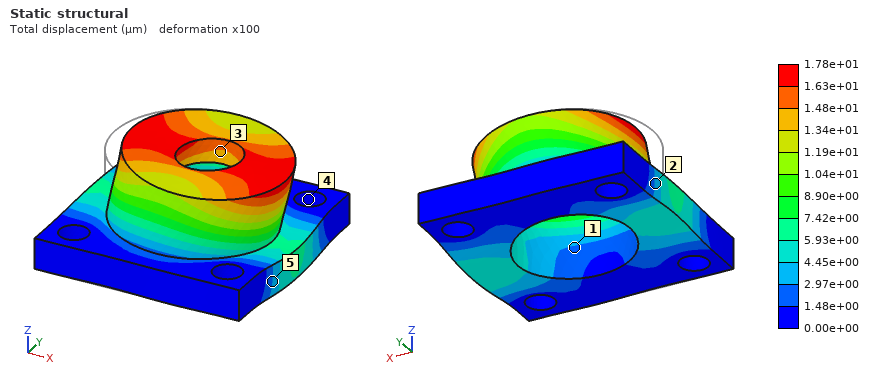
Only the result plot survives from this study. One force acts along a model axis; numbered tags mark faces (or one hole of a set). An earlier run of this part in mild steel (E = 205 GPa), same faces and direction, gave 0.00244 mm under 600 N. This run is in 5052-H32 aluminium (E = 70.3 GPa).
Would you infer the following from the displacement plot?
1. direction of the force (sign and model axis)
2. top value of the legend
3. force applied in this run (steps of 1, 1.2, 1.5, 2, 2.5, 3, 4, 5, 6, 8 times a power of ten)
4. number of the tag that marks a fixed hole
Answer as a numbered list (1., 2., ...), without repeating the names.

1. +X
2. 1.78e+01 µm
3. 1.5 kN
4. 4
